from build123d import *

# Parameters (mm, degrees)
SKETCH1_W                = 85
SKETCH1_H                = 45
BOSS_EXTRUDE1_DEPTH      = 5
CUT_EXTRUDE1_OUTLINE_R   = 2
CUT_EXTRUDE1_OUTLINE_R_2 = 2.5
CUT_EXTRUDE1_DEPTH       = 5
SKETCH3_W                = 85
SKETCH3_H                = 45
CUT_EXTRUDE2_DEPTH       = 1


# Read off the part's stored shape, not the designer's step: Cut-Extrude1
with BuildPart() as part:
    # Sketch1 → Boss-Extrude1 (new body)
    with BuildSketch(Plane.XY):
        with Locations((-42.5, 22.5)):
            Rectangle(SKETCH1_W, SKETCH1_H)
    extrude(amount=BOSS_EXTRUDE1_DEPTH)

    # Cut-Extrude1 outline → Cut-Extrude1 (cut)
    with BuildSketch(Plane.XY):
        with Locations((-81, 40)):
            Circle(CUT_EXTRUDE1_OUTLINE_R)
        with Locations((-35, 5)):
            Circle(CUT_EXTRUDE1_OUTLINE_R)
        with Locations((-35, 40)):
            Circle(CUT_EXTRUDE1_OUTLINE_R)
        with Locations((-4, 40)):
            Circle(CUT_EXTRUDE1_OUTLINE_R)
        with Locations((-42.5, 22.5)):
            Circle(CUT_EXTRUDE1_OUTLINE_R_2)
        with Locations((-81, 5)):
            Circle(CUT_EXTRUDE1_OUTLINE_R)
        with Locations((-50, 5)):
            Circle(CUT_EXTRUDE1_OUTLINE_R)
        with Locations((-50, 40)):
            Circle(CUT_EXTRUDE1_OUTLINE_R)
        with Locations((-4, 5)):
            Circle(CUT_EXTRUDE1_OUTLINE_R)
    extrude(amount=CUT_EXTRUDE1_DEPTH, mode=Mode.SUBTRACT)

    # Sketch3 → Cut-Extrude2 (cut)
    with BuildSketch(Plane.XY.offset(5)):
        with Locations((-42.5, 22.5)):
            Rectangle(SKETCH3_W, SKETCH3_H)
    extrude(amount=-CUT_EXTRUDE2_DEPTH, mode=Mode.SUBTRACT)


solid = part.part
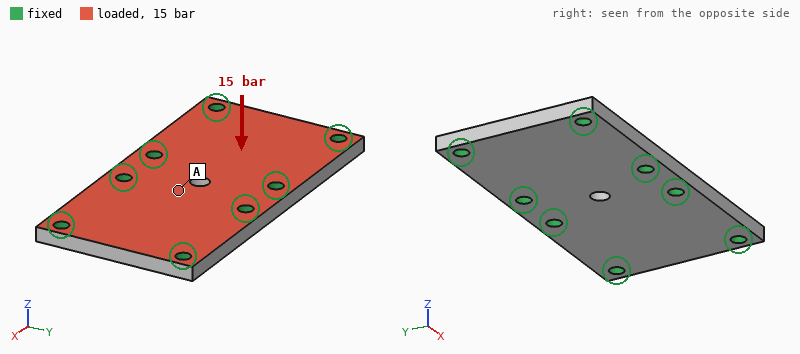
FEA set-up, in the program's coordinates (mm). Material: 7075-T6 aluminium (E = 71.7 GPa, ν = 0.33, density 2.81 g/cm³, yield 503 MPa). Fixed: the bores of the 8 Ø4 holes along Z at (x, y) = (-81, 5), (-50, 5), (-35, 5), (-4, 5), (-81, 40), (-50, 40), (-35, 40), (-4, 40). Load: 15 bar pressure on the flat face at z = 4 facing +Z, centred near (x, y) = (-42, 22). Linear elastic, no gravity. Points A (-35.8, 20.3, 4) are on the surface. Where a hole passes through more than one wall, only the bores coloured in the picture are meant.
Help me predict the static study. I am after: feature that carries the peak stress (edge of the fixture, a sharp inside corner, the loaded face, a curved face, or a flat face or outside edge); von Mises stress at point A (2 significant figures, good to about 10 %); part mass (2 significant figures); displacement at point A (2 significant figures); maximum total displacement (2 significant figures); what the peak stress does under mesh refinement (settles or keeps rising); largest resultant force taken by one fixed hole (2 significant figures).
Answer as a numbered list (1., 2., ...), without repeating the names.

1. edge of the fixture
2. 30 MPa
3. 42 g
4. 19 µm
5. 28 µm
6. keeps rising
7. 760 N
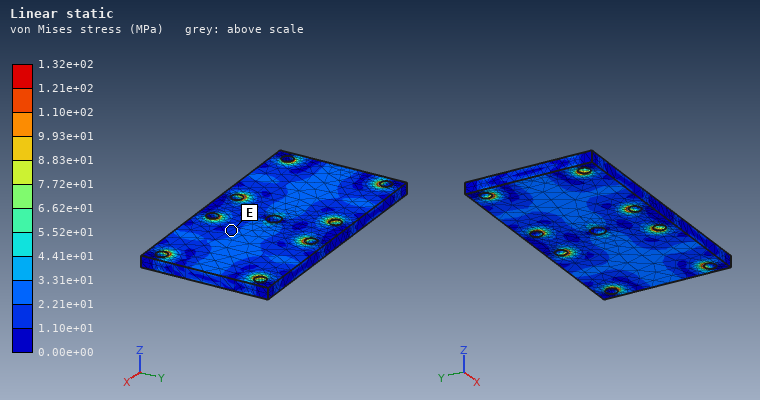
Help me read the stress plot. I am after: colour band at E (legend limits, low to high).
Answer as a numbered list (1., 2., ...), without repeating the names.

1. 1.10e+01 to 2.21e+01 MPa
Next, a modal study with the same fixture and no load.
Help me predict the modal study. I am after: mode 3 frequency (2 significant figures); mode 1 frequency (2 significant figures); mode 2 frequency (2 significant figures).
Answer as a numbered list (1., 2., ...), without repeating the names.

1. 19 kHz
2. 13 kHz
3. 13 kHz
